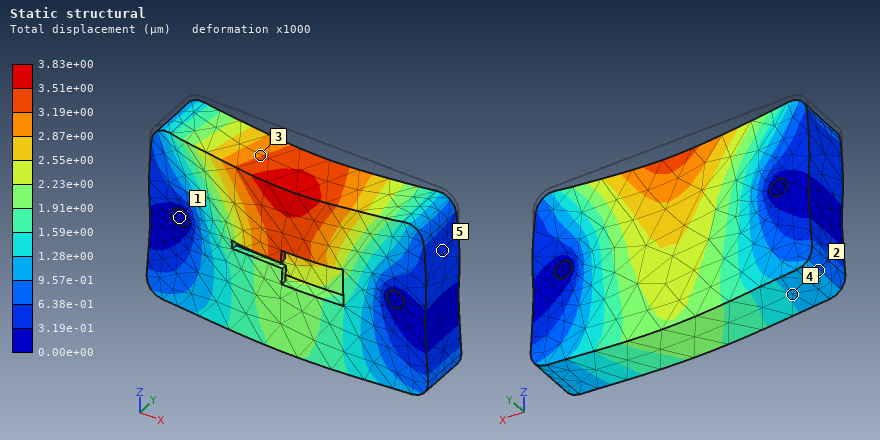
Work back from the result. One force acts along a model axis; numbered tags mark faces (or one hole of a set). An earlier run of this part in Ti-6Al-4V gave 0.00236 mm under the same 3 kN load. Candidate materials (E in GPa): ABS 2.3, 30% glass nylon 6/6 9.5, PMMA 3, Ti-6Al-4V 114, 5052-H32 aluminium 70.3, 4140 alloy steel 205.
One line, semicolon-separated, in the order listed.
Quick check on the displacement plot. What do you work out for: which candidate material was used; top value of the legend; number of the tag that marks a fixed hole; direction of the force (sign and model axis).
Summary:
5052-H32 aluminium; 3.83e+00 µm; 1; -Z
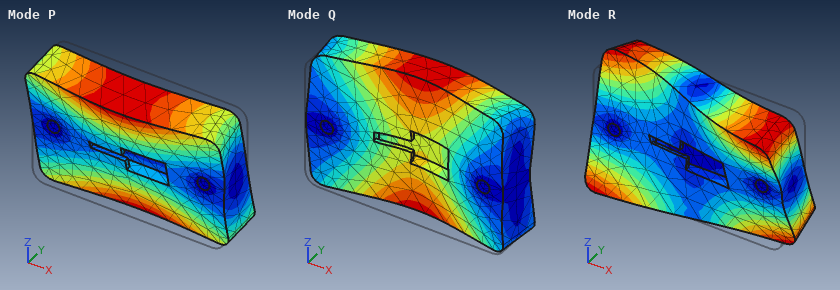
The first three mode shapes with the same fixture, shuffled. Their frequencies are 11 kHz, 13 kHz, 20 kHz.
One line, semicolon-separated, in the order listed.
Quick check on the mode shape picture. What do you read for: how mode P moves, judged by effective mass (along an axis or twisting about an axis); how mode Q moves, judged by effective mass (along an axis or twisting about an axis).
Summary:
twisting about X; along Y
